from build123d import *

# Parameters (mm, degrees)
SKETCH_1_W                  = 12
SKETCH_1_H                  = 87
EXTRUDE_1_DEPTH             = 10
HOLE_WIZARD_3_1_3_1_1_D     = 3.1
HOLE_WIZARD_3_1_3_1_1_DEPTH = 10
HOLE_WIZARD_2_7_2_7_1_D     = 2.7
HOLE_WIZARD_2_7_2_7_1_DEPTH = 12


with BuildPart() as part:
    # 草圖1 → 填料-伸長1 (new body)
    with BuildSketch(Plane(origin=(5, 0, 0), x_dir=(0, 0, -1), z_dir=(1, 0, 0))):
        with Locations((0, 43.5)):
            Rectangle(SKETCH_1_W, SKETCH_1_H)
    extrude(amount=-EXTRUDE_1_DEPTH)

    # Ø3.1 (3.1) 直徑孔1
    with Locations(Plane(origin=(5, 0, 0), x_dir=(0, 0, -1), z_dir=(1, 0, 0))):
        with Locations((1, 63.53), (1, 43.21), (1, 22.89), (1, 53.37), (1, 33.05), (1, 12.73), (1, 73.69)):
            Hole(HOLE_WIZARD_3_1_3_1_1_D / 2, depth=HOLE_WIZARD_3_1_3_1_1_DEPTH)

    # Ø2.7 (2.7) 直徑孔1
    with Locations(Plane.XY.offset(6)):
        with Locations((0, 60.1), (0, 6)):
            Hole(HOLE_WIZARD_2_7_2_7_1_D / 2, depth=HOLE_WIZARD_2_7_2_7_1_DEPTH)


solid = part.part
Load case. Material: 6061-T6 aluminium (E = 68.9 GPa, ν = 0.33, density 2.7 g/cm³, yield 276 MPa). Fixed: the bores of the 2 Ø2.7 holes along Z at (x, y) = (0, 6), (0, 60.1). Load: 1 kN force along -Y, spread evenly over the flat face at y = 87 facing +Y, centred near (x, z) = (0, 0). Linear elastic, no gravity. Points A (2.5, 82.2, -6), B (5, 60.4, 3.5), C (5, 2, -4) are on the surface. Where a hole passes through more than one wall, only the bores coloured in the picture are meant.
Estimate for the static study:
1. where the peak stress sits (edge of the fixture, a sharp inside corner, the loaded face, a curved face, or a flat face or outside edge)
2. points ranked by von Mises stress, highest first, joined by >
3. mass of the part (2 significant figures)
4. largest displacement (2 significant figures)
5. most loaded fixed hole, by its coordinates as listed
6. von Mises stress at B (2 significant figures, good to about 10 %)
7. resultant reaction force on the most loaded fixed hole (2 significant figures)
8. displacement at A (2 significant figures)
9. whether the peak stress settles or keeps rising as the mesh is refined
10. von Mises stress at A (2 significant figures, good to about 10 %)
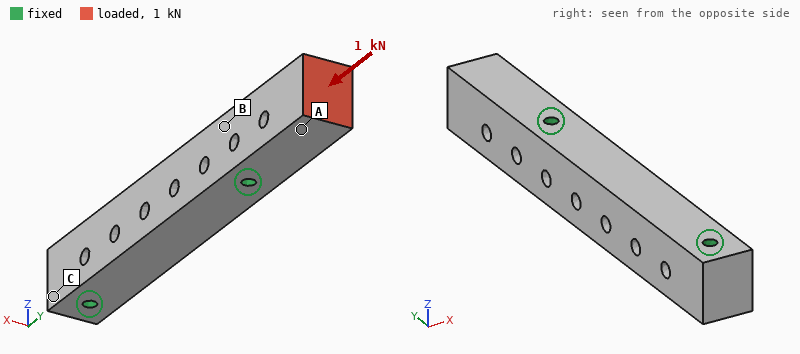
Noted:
edge of the fixture
A > B > C
26 g
4.1 µm
(0, 60.1)
5.1 MPa
970 N
3.5 µm
keeps rising
8.8 MPa
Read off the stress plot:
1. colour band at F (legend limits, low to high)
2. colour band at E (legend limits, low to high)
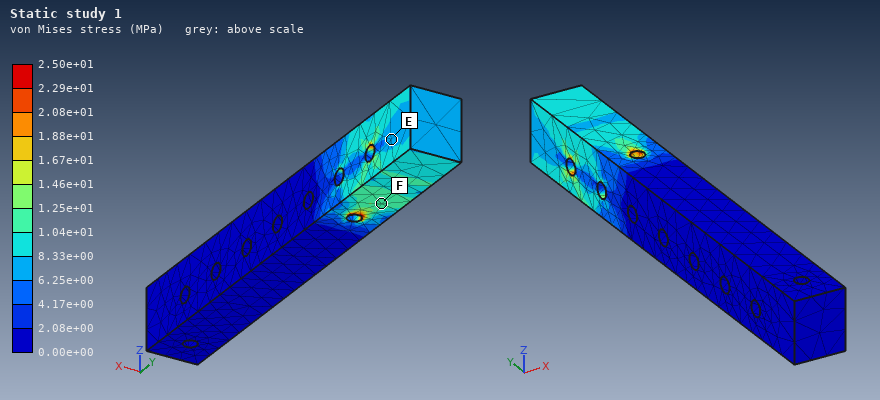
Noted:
1.04e+01 to 1.25e+01 MPa
6.25e+00 to 8.33e+00 MPa
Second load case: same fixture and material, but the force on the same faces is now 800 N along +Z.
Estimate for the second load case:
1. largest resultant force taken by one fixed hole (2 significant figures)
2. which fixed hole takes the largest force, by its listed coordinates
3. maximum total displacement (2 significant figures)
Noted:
840 N
(0, 60.1)
70 µm
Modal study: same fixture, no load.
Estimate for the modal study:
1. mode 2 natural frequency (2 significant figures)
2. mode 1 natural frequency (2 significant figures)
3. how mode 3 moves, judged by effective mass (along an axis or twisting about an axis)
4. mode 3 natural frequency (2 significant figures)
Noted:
11 kHz
7300 Hz
along X
12 kHz
